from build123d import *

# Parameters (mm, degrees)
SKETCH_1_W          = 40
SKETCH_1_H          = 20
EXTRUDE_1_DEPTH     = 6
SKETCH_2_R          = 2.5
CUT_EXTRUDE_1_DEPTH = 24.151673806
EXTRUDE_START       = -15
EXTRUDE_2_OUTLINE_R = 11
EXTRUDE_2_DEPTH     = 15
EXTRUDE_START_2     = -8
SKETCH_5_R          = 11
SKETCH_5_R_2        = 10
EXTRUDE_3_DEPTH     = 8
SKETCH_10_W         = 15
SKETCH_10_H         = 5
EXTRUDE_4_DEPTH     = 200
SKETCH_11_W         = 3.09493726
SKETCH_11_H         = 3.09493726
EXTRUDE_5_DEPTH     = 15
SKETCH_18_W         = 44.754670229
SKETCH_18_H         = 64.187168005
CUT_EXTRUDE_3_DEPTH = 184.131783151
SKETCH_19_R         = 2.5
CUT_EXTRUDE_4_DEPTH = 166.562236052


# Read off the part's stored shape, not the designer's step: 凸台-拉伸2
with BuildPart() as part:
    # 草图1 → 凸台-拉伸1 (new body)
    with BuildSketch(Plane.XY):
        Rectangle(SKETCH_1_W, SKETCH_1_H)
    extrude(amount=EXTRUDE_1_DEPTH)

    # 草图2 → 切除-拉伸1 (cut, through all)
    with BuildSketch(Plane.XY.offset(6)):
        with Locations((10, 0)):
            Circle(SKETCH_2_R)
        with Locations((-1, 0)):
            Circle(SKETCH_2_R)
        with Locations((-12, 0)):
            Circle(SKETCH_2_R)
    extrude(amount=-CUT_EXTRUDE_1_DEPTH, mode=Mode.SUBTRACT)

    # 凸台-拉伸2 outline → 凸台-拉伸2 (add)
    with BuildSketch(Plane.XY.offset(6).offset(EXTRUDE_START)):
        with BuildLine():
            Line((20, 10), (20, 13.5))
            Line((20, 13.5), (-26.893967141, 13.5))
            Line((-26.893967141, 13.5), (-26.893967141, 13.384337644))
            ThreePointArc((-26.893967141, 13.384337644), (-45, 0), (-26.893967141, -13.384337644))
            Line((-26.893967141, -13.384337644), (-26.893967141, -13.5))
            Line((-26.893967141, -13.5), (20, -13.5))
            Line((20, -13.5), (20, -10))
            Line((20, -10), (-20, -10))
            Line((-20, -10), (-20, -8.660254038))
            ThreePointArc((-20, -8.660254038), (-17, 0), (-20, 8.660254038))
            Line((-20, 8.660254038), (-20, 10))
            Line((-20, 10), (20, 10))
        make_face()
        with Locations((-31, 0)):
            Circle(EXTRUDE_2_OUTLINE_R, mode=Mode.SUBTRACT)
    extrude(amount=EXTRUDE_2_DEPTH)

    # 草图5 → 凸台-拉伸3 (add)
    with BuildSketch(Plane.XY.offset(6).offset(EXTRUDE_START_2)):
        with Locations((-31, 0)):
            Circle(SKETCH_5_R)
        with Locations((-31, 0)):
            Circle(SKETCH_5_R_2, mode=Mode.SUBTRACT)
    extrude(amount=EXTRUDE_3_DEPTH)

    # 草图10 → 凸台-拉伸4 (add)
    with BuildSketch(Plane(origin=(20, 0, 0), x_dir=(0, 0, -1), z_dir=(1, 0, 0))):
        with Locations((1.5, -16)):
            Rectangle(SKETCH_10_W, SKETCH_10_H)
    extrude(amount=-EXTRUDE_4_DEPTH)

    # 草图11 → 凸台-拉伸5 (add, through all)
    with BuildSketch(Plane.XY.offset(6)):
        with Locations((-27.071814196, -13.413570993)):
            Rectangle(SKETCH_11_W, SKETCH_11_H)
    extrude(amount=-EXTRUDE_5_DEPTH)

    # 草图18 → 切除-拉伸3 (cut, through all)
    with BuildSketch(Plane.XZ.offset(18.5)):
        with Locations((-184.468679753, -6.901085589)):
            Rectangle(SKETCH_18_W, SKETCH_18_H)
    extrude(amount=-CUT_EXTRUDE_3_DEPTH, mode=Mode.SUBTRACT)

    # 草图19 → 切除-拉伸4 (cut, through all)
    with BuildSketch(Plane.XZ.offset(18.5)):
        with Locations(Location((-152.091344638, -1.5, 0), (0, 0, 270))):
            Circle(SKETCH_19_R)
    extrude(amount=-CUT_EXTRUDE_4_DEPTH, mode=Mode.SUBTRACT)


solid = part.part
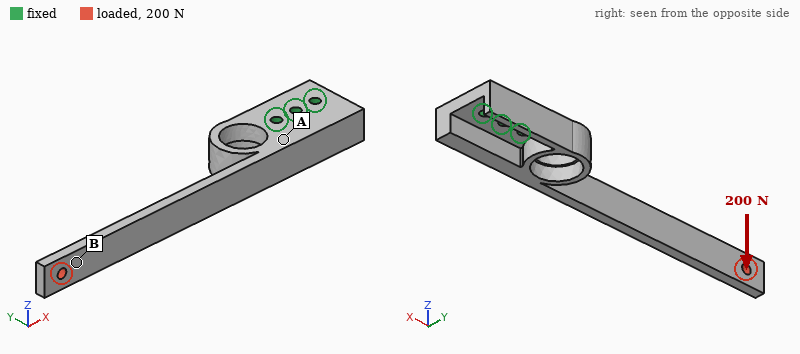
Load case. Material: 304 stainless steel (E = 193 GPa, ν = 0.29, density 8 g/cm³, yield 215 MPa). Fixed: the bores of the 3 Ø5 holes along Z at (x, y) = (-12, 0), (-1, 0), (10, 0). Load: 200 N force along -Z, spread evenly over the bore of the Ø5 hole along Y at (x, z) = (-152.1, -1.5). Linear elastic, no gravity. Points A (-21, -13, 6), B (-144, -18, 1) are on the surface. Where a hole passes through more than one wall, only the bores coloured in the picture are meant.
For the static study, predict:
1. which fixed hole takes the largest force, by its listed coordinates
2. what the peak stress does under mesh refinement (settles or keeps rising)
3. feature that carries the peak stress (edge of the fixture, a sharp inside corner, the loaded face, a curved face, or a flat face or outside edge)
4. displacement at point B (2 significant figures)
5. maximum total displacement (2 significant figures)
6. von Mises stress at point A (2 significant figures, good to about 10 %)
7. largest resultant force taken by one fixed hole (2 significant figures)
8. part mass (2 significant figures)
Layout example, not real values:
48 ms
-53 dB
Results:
(-12, 0)
keeps rising
edge of the fixture
0.56 mm
0.69 mm
55 MPa
1.2 kN
210 g
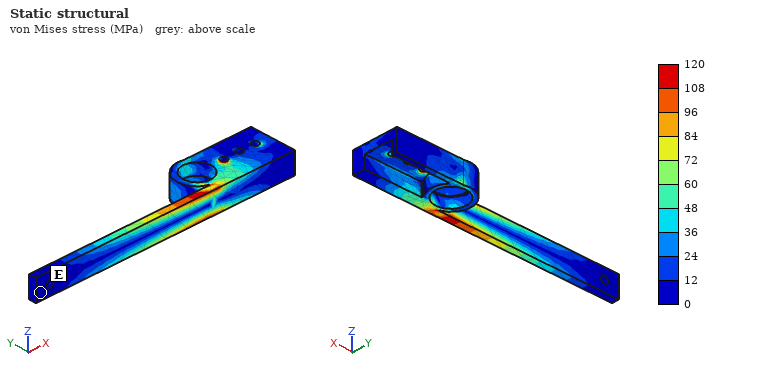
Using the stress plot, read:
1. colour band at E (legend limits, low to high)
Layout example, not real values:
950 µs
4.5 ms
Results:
0 to 12 MPa
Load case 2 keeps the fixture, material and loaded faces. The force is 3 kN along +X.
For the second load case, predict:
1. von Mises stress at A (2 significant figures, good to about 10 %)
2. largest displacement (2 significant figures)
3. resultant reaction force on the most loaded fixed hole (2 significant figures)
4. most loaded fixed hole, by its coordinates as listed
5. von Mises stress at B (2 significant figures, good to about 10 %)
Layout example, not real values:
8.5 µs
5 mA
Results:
20 MPa
0.11 mm
2.2 kN
(-12, 0)
42 MPa
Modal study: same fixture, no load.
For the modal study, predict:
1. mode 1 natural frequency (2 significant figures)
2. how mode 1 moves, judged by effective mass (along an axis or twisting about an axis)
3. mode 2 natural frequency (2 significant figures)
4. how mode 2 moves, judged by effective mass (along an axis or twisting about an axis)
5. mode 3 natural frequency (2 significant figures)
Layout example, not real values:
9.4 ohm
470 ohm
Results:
230 Hz
along Y
560 Hz
along Z
1400 Hz
